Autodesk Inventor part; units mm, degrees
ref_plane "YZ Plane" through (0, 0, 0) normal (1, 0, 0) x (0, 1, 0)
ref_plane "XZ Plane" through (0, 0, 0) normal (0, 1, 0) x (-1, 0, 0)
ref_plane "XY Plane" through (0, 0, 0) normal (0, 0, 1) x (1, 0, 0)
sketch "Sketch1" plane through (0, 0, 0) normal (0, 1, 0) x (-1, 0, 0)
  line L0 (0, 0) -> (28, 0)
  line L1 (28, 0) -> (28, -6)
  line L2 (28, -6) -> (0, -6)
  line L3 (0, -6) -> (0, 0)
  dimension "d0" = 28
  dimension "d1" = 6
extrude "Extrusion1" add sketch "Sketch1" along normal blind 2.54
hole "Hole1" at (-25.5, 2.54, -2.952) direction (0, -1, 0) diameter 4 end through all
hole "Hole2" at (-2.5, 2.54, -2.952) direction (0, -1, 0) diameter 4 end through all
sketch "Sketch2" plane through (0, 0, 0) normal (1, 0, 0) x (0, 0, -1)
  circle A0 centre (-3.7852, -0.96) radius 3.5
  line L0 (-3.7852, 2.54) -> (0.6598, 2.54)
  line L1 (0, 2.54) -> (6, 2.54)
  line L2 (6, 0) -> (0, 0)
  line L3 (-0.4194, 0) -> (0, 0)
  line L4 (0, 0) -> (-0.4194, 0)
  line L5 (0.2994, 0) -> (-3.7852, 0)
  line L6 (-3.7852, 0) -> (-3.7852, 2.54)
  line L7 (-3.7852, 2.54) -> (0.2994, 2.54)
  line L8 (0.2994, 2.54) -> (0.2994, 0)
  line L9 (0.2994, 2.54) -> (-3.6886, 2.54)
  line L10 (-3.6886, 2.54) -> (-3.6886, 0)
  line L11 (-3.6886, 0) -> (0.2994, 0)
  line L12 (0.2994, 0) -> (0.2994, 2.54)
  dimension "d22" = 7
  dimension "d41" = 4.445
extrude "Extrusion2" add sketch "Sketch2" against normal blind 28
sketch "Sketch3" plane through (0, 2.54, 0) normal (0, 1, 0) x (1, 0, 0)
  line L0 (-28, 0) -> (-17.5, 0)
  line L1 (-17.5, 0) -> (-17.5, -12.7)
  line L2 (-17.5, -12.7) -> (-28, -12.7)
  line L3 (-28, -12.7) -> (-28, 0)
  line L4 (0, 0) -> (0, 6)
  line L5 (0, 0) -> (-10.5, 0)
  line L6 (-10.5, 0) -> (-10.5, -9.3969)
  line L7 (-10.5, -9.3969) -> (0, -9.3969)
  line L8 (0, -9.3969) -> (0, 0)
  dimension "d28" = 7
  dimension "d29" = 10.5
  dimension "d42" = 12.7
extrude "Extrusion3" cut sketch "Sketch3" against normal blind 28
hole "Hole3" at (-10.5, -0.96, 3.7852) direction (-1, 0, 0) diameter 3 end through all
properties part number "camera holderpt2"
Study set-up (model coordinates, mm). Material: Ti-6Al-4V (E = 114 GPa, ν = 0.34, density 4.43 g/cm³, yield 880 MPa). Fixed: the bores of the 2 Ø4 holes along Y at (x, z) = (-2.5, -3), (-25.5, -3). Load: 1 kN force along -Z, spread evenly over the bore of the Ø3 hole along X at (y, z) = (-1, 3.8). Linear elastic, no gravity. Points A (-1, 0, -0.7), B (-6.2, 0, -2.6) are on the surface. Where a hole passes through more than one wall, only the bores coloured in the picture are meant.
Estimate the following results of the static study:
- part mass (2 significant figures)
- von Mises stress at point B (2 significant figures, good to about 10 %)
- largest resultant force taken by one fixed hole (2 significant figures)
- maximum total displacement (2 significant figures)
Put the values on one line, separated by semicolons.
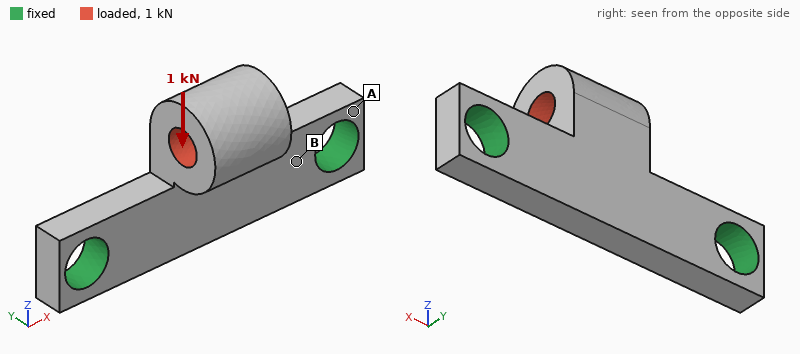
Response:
2.7 g; 240 MPa; 510 N; 0.14 mm
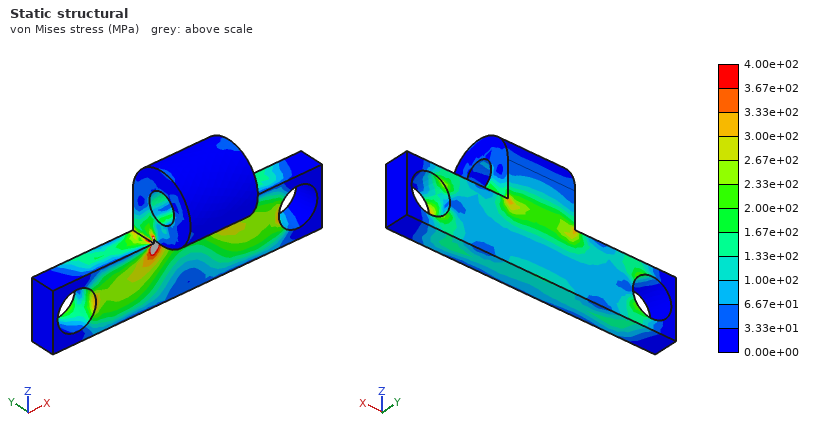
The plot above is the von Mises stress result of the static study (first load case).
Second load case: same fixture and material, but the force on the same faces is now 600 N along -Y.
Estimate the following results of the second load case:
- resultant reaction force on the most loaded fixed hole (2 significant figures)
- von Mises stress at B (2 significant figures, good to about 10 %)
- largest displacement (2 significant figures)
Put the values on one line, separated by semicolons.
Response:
300 N; 320 MPa; 0.23 mm
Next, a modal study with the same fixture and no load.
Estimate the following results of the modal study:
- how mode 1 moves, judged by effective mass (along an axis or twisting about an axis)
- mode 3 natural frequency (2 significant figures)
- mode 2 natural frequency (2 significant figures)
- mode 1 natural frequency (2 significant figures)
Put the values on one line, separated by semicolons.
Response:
along Y; 26 kHz; 26 kHz; 8900 Hz
